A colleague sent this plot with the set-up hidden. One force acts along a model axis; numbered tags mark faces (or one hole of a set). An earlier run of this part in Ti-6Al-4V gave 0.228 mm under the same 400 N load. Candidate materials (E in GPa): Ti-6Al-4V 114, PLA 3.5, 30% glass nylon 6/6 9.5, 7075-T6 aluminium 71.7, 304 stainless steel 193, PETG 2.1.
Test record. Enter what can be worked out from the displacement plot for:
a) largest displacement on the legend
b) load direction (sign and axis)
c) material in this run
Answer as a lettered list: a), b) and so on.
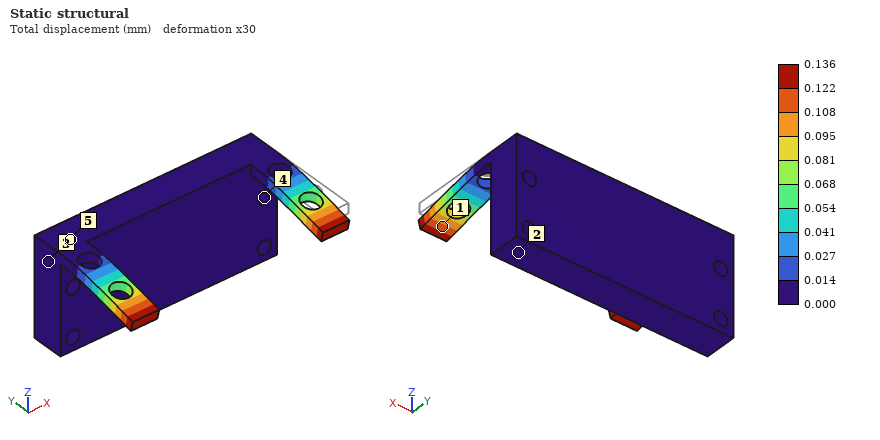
a) 0.136 mm
b) -Z
c) 304 stainless steel
